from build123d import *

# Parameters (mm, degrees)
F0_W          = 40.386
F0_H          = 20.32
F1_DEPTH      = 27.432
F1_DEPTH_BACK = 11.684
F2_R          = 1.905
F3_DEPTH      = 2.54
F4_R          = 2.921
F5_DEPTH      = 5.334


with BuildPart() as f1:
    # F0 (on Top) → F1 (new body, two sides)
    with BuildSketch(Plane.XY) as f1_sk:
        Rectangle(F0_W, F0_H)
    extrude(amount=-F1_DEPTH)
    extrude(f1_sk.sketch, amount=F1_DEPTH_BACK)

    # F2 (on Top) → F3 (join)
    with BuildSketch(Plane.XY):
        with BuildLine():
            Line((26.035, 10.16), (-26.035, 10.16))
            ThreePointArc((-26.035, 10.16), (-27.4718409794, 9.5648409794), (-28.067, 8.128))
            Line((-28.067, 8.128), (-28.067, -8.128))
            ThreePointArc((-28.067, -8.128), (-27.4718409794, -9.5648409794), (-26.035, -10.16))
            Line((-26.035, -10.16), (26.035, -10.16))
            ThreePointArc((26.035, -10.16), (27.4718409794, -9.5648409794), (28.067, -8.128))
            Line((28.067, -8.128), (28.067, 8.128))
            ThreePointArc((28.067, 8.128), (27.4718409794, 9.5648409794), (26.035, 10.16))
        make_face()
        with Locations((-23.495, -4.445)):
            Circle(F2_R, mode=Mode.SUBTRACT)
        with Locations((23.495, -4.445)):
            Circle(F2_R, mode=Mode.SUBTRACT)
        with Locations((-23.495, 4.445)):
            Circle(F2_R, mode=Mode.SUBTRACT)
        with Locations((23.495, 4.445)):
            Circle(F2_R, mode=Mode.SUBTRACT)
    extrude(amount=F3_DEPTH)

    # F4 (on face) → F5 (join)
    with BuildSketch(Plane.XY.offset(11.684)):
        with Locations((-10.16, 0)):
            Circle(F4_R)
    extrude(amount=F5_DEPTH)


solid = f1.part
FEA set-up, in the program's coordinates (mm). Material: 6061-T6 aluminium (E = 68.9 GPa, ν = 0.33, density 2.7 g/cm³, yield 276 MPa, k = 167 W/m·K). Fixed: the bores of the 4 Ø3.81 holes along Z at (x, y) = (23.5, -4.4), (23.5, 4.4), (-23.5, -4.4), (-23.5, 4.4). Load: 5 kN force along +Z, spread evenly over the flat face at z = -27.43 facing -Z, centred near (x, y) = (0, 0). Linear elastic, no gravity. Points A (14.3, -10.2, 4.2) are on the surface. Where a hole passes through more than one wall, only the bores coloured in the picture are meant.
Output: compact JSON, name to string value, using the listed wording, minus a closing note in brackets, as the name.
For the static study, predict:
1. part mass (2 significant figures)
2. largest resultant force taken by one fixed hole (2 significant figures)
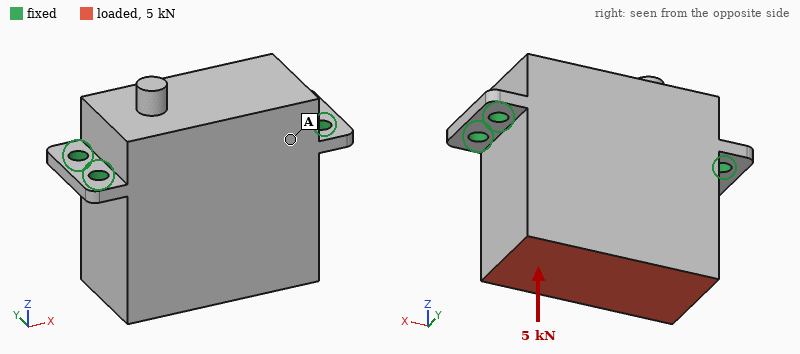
{"part mass": "89 g", "largest resultant force taken by one fixed hole": "1.3 kN"}
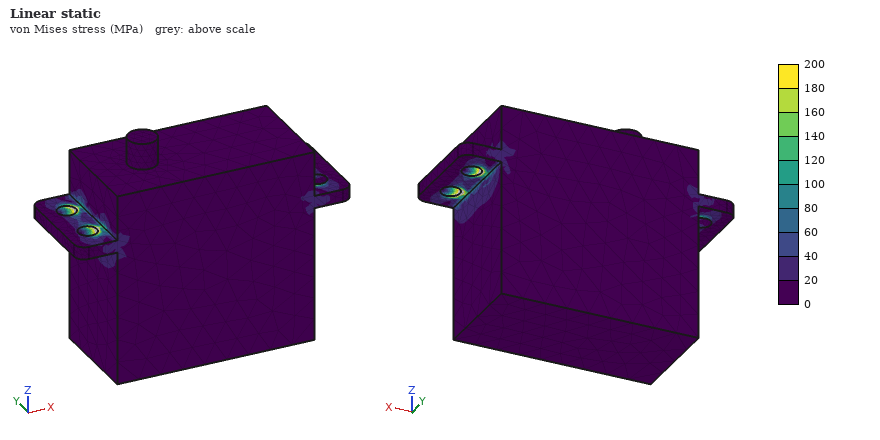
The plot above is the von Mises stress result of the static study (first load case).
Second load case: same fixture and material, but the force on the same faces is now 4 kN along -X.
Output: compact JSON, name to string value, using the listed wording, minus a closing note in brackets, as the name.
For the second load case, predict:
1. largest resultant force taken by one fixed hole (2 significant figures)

{"largest resultant force taken by one fixed hole": "1.7 kN"}
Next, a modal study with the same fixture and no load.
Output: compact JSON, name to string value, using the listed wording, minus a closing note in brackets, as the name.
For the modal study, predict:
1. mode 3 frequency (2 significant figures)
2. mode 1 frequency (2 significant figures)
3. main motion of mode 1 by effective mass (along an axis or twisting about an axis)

{"mode 3 frequency": "11 kHz", "mode 1 frequency": "3600 Hz", "main motion of mode 1 by effective mass": "along Y"}
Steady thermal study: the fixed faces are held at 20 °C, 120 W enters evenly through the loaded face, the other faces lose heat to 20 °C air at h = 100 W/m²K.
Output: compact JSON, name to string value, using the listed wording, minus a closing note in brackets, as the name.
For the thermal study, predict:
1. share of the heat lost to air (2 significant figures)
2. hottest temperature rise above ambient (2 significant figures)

{"share of the heat lost to air": "16 %", "hottest temperature rise above ambient": "50 K"}
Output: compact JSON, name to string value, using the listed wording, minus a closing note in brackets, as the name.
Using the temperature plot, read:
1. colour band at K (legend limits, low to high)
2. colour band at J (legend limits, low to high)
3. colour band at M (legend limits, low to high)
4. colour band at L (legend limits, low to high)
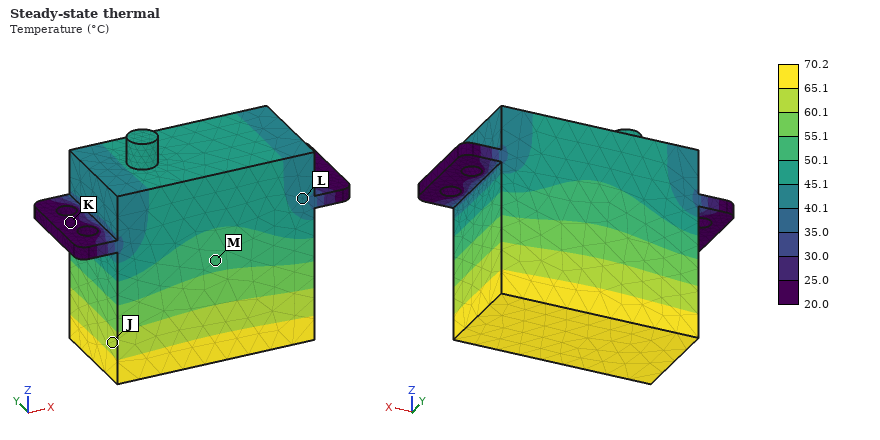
{"colour band at K": "20.0 to 25.0 °C", "colour band at J": "60.1 to 65.1 °C", "colour band at M": "50.1 to 55.1 °C", "colour band at L": "40.1 to 45.1 °C"}
